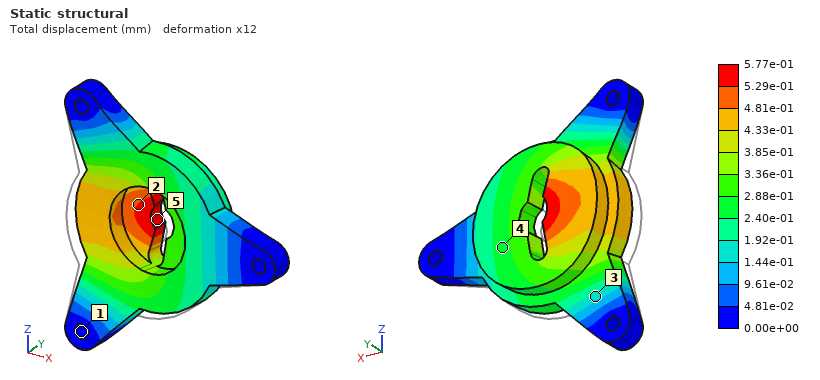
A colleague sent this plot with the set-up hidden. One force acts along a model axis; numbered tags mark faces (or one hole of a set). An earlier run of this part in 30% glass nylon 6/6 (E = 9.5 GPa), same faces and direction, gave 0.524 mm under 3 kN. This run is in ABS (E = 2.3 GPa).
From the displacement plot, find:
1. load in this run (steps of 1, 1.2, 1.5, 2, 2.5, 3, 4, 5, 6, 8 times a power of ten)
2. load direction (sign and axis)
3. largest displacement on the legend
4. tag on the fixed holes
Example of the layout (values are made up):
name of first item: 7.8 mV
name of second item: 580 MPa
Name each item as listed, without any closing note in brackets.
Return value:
load in this run: 800 N
load direction: +Y
largest displacement on the legend: 5.77e-01 mm
tag on the fixed holes: 1
